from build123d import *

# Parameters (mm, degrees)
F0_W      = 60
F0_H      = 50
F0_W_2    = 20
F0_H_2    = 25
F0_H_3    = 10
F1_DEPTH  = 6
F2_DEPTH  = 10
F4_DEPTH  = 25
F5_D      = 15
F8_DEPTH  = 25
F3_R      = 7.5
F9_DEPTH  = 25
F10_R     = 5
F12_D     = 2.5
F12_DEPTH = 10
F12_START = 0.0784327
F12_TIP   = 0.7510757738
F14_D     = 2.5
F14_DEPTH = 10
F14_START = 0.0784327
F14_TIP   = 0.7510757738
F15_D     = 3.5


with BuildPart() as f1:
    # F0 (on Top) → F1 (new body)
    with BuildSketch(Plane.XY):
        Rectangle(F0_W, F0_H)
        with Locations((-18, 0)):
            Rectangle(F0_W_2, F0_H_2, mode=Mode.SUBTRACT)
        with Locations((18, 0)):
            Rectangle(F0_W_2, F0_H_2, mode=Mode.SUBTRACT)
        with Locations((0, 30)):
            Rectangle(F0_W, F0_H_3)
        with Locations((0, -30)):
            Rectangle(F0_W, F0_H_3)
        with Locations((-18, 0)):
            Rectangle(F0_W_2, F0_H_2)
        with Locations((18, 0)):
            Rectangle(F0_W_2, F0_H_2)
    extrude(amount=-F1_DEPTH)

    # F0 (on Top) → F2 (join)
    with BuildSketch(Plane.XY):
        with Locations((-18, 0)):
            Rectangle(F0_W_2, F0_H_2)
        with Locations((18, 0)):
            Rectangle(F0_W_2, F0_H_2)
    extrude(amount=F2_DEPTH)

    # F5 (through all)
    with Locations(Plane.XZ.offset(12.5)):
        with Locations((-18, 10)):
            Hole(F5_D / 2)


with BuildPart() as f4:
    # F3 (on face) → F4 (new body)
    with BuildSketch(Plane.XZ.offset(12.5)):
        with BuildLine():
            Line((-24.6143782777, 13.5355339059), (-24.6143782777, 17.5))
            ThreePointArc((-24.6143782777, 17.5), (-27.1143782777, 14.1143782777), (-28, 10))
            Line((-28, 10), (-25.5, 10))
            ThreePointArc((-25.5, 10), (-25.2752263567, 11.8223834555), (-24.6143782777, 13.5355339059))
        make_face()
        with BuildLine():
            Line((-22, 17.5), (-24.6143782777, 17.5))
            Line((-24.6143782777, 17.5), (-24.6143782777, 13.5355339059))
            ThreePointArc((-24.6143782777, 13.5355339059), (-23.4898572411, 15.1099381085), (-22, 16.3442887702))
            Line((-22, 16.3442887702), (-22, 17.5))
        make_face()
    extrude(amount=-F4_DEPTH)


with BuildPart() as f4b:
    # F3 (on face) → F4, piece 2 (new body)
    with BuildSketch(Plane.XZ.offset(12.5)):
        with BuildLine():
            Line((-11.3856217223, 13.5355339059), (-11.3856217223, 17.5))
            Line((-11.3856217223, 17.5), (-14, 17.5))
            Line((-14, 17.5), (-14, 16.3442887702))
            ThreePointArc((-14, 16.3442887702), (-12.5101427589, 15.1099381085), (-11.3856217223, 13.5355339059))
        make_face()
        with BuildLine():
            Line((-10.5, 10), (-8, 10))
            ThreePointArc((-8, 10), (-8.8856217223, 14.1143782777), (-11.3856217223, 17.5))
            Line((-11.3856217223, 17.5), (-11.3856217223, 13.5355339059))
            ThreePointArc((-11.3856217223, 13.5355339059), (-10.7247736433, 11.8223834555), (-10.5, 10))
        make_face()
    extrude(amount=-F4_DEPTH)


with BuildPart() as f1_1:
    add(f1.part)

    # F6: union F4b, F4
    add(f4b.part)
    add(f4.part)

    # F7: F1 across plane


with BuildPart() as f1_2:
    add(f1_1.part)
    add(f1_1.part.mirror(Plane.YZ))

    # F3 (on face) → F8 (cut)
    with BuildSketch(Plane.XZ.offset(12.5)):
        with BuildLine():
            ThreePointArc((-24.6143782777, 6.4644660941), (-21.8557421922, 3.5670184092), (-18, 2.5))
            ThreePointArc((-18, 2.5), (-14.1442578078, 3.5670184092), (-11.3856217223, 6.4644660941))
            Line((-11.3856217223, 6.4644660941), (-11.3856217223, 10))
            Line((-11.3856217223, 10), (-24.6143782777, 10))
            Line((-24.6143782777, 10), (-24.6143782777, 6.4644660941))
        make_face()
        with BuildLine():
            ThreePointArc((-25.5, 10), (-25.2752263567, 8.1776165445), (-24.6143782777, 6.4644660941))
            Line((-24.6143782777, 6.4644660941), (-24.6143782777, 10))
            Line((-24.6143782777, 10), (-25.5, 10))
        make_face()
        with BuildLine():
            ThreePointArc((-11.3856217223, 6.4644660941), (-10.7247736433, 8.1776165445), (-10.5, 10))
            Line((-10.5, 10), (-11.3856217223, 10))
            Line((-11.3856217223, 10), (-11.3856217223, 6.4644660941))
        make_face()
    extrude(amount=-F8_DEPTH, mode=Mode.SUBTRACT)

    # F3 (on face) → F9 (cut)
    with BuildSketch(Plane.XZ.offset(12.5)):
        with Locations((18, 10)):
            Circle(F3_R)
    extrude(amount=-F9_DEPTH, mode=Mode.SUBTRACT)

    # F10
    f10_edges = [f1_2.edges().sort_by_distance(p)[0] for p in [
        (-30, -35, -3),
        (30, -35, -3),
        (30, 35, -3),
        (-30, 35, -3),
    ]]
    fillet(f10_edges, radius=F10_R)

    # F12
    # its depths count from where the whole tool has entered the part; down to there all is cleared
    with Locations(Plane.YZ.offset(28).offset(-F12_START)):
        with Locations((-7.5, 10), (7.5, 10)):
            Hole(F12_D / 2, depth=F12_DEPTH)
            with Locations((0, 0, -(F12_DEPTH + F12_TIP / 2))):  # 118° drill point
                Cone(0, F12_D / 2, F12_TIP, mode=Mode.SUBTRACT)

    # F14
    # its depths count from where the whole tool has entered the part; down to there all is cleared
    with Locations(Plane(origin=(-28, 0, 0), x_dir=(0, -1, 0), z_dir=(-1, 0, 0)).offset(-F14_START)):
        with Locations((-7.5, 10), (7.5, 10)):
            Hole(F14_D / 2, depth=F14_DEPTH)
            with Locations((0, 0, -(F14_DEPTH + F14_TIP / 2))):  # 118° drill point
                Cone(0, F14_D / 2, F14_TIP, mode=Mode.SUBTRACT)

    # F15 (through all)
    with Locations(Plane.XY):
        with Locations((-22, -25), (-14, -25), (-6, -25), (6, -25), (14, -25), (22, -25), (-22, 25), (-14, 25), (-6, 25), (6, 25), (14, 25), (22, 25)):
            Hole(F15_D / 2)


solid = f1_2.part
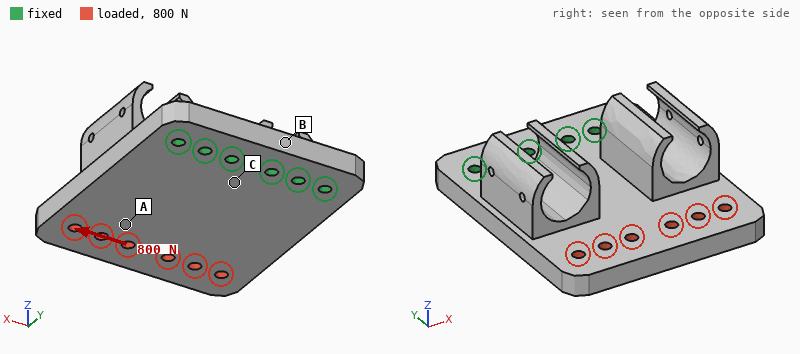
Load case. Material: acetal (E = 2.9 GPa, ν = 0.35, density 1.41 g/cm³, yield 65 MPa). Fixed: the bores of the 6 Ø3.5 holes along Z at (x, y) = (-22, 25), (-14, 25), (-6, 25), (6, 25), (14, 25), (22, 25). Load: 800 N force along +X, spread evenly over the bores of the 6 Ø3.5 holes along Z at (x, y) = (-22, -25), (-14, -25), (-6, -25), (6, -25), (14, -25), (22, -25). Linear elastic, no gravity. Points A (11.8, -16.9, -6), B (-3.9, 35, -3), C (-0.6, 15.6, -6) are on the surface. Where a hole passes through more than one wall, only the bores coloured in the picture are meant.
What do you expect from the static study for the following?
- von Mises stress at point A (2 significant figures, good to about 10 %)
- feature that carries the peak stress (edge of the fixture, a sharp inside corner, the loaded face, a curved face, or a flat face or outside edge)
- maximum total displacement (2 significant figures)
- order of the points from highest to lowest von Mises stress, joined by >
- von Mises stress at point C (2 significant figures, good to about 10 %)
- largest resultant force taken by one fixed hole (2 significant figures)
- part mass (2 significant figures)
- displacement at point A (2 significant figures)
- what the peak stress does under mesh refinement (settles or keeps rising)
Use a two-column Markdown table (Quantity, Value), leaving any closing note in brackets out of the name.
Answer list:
| Quantity | Value |
|---|---|
| von Mises stress at point A | 4.7 MPa |
| feature that carries the peak stress | edge of the fixture |
| maximum total displacement | 0.30 mm |
| order of the points from highest to lowest von Mises stress, joined by > | C > A > B |
| von Mises stress at point C | 7.0 MPa |
| largest resultant force taken by one fixed hole | 730 N |
| part mass | 45 g |
| displacement at point A | 0.20 mm |
| what the peak stress does under mesh refinement | keeps rising |
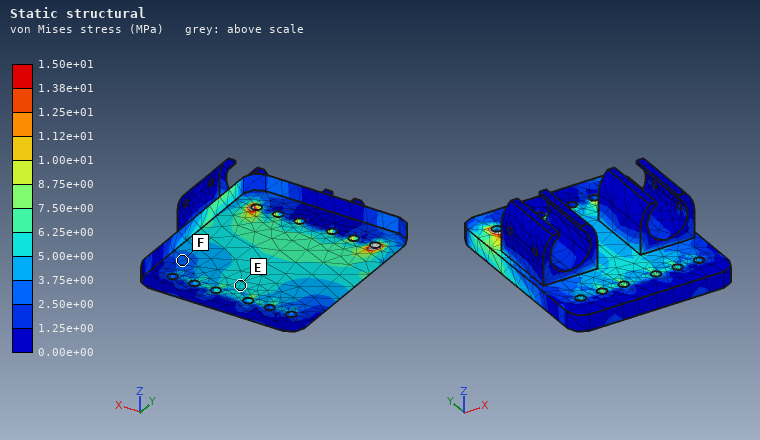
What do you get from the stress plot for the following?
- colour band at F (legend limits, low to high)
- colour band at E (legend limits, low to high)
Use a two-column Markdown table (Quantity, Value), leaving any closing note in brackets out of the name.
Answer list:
| Quantity | Value |
|---|---|
| colour band at F | 2.50e+00 to 3.75e+00 MPa |
| colour band at E | 5.00e+00 to 6.25e+00 MPa |
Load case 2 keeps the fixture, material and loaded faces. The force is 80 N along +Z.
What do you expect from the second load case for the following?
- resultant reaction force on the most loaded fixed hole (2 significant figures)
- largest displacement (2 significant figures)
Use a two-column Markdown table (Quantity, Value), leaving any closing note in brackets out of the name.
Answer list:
| Quantity | Value |
|---|---|
| resultant reaction force on the most loaded fixed hole | 23 N |
| largest displacement | 0.94 mm |
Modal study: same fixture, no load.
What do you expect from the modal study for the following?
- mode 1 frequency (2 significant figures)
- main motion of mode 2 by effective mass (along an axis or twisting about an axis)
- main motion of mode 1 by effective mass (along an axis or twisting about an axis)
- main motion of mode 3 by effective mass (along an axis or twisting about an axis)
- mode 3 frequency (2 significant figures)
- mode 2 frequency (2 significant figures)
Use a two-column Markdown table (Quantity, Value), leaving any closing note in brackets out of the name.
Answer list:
| Quantity | Value |
|---|---|
| mode 1 frequency | 430 Hz |
| main motion of mode 2 by effective mass | twisting about Y |
| main motion of mode 1 by effective mass | along Z |
| main motion of mode 3 by effective mass | along X |
| mode 3 frequency | 2200 Hz |
| mode 2 frequency | 970 Hz |
